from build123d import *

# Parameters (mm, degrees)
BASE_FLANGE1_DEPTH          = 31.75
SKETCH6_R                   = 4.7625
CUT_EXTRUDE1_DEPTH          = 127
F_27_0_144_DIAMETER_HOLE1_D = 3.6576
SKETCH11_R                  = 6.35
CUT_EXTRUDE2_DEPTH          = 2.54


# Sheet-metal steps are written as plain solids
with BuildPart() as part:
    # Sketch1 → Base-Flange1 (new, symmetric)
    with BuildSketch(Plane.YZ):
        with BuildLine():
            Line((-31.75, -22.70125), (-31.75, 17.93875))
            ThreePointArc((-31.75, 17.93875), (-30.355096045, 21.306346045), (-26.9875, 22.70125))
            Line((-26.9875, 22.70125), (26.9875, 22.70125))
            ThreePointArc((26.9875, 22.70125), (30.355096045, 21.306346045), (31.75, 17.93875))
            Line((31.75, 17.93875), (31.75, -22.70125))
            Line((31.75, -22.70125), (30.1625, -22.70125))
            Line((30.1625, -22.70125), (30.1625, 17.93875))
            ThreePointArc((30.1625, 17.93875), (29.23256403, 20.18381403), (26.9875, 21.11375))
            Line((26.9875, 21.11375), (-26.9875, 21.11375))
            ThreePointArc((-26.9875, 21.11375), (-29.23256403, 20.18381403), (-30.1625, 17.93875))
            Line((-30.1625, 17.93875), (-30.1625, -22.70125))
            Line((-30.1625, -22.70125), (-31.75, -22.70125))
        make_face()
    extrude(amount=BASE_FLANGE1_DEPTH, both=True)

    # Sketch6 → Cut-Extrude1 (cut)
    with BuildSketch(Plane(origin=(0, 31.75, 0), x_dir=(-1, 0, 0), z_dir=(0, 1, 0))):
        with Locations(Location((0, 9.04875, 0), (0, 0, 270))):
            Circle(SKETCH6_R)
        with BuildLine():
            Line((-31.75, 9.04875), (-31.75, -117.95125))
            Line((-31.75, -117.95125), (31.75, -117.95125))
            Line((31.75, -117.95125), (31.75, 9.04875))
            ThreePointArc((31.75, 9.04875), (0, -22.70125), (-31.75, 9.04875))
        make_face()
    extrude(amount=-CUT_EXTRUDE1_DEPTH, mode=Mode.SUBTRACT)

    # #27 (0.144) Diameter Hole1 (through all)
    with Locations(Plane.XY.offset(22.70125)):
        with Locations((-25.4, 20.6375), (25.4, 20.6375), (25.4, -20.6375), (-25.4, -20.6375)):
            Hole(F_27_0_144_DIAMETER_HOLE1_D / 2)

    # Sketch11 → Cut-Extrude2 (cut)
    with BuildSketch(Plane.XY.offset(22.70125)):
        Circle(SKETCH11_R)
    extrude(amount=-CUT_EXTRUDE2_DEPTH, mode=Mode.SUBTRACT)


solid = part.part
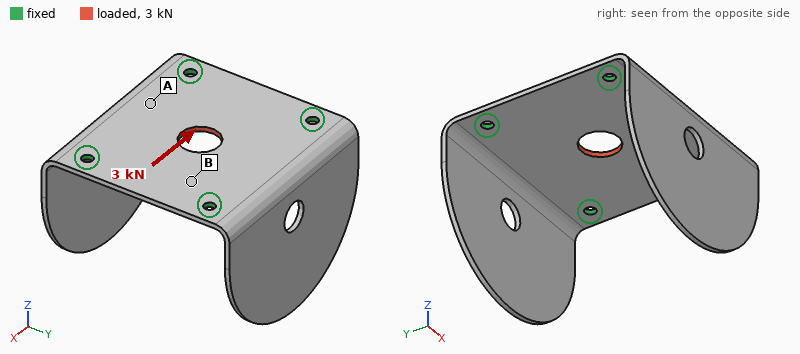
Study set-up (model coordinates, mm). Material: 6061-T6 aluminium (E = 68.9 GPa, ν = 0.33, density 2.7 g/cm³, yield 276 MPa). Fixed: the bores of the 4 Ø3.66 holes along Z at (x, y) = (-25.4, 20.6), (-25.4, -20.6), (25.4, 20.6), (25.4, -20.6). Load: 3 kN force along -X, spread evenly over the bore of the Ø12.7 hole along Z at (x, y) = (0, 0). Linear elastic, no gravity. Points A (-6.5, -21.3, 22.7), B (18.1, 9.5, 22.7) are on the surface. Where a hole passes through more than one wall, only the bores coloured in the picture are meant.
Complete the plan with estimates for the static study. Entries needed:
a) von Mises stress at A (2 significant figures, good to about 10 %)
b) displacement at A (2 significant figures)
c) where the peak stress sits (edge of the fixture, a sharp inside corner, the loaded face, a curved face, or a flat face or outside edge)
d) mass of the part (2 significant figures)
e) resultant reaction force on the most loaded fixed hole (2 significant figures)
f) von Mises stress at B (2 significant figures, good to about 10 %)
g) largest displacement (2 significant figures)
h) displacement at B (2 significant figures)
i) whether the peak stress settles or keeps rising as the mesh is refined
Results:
12 MPa
5.4 µm
edge of the fixture
35 g
810 N
30 MPa
18 µm
9.5 µm
keeps rising
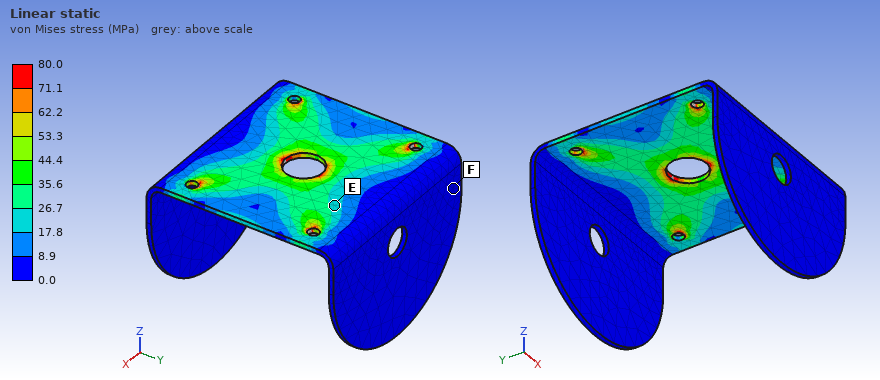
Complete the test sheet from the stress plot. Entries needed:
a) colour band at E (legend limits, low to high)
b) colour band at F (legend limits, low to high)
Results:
17.8 to 26.7 MPa
0.0 to 8.9 MPa
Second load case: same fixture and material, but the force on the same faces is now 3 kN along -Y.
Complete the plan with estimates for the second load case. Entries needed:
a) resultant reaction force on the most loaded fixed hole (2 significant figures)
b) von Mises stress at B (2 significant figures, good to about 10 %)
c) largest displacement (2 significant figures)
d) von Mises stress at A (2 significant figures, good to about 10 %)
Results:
790 N
30 MPa
21 µm
18 MPa
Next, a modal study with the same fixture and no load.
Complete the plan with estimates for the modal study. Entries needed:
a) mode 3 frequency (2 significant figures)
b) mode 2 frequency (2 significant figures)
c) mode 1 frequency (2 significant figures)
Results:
1500 Hz
600 Hz
590 Hz
